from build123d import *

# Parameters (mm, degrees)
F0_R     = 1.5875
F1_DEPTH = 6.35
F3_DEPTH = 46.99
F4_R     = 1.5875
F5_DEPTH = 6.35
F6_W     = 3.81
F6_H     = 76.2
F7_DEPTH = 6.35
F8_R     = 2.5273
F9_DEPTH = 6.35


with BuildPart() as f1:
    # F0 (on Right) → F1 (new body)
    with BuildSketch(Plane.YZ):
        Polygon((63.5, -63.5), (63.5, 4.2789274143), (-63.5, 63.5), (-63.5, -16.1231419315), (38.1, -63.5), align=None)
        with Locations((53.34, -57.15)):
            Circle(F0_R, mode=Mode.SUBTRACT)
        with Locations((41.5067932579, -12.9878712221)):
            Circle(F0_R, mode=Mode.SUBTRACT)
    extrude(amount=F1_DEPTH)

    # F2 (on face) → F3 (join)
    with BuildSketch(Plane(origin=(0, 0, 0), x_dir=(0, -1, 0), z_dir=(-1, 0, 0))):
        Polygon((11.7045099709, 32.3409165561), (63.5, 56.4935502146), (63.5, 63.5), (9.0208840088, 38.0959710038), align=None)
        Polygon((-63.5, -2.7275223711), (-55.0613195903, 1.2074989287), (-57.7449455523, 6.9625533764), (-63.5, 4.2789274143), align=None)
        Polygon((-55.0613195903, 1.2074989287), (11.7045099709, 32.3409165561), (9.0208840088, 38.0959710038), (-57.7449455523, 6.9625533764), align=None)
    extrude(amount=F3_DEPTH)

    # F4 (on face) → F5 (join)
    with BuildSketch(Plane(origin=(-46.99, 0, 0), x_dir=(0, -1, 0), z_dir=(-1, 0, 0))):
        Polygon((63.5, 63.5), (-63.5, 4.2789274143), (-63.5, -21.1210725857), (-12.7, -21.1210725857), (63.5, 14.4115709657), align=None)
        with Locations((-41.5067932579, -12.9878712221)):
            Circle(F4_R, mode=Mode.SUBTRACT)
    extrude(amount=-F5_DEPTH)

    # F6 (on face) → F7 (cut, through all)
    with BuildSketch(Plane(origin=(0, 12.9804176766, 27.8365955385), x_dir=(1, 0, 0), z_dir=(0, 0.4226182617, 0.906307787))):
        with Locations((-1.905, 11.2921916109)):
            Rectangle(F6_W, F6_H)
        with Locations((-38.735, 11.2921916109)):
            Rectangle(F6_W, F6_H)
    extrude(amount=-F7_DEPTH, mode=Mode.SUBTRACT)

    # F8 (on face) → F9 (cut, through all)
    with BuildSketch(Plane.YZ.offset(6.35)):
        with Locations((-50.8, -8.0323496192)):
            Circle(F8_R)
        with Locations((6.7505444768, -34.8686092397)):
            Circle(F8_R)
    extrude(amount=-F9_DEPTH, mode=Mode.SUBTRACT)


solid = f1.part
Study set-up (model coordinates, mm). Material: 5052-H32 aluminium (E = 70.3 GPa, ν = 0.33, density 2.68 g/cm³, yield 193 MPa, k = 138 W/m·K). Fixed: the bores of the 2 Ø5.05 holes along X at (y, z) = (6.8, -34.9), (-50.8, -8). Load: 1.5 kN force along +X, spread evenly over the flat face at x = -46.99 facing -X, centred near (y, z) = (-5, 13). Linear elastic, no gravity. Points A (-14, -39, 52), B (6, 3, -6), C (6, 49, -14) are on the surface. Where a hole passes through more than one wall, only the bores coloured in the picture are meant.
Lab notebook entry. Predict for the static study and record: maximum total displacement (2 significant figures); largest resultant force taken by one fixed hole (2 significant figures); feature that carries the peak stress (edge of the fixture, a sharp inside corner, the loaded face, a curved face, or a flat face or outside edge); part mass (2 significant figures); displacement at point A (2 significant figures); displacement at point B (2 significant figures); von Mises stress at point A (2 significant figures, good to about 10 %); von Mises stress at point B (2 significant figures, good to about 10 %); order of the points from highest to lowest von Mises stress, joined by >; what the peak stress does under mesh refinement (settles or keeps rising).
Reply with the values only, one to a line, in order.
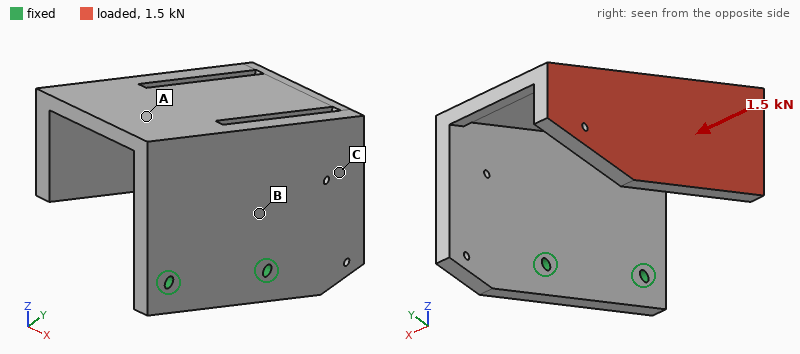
0.80 mm
790 N
edge of the fixture
350 g
0.36 mm
0.12 mm
38 MPa
27 MPa
A > B > C
keeps rising
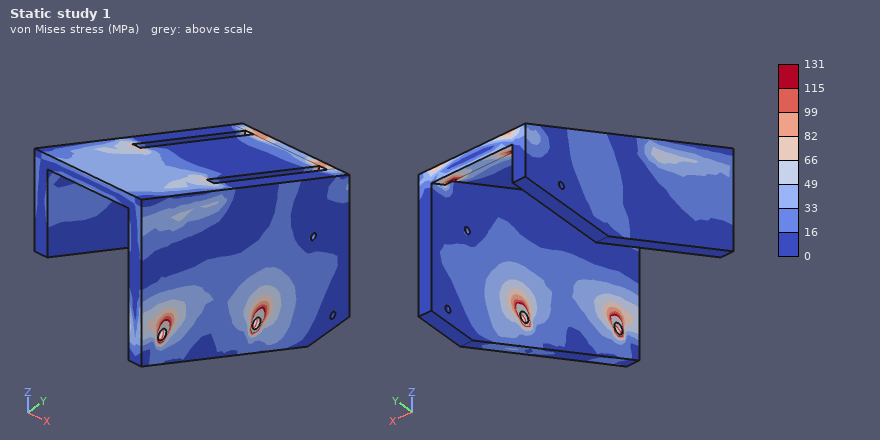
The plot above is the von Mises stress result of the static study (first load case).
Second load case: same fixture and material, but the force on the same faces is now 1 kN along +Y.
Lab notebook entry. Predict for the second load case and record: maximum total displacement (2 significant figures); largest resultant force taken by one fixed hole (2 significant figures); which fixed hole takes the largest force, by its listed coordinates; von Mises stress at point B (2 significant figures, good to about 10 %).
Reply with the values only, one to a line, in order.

0.93 mm
1.0 kN
(-50.8, -8)
32 MPa
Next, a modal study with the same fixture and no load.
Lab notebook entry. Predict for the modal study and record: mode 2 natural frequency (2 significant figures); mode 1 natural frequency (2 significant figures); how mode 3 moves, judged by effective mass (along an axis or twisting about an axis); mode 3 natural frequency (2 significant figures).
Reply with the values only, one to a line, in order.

570 Hz
370 Hz
along X
690 Hz
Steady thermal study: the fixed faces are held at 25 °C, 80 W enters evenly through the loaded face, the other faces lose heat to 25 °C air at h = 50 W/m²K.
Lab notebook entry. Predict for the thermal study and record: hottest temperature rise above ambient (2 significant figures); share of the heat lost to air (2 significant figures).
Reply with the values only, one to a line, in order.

76 K
70 %
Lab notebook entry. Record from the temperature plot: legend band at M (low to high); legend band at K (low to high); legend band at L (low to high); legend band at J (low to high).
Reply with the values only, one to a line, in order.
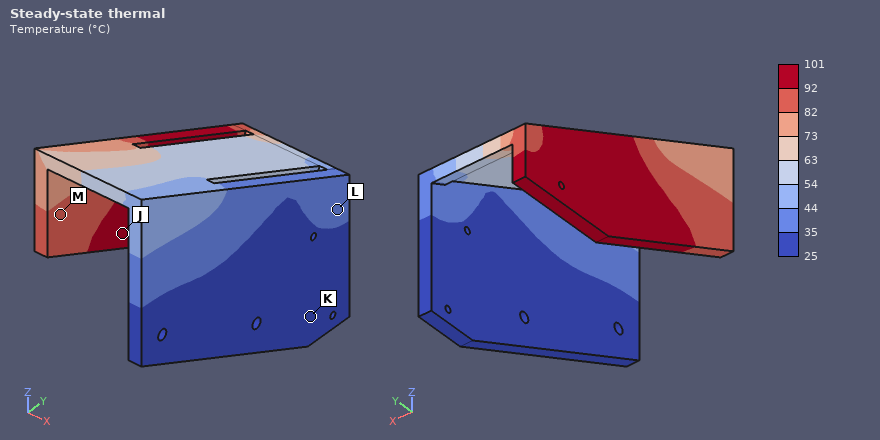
82 to 92 °C
25 to 35 °C
35 to 44 °C
92 to 101 °C
